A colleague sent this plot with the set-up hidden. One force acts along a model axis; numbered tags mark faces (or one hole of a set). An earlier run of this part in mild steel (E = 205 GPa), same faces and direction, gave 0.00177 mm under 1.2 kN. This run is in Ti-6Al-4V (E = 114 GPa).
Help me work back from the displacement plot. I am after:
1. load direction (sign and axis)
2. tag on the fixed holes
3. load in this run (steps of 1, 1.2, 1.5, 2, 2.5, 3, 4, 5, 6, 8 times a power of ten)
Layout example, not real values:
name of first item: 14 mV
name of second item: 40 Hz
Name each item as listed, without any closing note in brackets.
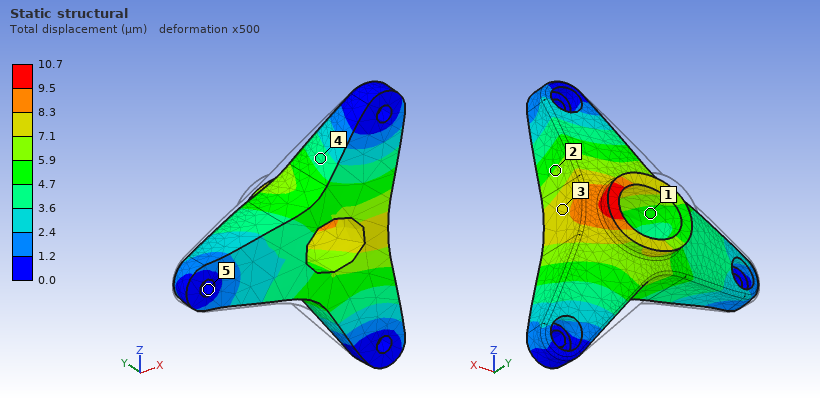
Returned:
load direction: +X
tag on the fixed holes: 5
load in this run: 4 kN
